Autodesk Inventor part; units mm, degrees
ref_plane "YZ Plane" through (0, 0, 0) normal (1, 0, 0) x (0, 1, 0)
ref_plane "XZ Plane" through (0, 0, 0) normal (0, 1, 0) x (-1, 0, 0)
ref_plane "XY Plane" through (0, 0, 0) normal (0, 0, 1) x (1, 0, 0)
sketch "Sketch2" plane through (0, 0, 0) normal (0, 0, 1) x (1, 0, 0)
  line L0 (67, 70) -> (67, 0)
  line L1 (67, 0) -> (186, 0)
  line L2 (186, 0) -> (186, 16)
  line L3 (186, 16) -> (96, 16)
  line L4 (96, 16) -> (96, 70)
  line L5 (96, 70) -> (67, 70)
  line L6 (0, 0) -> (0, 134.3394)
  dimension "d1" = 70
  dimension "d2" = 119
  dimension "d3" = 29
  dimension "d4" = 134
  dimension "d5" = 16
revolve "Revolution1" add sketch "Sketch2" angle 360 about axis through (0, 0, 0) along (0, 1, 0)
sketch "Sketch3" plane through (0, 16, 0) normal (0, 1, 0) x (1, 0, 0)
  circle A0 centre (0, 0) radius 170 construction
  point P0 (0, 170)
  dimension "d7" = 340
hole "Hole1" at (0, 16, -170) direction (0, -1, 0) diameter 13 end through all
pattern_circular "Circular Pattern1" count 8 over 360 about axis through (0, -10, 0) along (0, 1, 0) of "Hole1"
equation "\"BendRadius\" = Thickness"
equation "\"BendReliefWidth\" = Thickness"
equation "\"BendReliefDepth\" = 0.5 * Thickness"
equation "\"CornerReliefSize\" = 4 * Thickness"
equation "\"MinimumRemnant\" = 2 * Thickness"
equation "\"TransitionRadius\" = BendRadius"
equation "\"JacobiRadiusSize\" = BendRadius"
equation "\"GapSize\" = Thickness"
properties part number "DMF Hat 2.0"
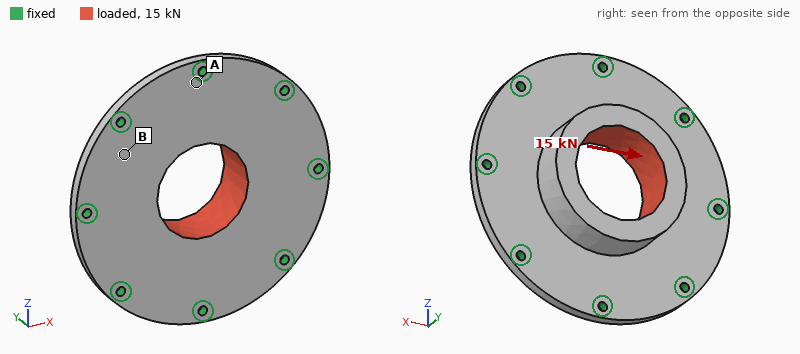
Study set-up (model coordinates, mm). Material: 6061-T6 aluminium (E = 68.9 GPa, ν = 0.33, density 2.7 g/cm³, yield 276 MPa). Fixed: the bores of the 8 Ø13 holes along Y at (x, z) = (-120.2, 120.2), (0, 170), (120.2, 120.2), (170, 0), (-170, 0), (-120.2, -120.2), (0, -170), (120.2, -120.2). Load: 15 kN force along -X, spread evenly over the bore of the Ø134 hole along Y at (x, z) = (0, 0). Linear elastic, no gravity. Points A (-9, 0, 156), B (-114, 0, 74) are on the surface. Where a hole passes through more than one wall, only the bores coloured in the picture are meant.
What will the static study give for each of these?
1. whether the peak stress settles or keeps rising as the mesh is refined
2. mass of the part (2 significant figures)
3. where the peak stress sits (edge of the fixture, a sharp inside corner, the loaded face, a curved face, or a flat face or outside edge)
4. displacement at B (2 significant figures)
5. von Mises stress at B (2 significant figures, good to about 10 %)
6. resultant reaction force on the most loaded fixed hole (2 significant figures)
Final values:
keeps rising
6.2 kg
edge of the fixture
6.8 µm
1.5 MPa
2.8 kN
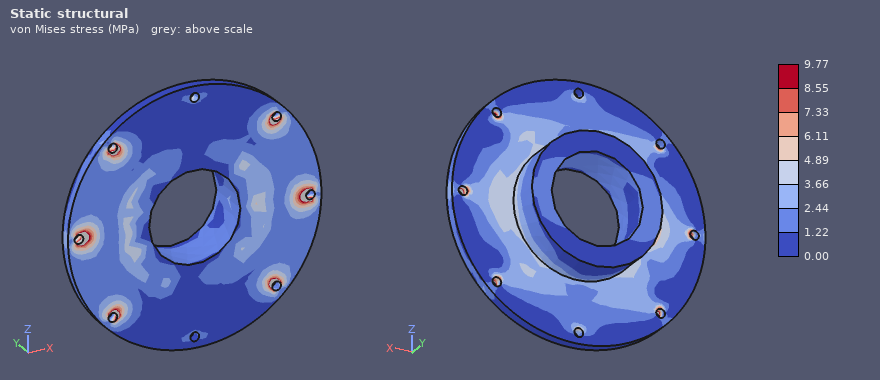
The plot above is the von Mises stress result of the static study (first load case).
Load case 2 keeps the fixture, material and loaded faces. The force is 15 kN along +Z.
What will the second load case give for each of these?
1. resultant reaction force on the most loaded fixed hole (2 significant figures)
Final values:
2.8 kN
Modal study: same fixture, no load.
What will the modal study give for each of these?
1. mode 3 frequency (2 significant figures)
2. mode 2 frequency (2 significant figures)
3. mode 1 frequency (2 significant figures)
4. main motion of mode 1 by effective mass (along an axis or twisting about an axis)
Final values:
2000 Hz
2000 Hz
1400 Hz
along Y
